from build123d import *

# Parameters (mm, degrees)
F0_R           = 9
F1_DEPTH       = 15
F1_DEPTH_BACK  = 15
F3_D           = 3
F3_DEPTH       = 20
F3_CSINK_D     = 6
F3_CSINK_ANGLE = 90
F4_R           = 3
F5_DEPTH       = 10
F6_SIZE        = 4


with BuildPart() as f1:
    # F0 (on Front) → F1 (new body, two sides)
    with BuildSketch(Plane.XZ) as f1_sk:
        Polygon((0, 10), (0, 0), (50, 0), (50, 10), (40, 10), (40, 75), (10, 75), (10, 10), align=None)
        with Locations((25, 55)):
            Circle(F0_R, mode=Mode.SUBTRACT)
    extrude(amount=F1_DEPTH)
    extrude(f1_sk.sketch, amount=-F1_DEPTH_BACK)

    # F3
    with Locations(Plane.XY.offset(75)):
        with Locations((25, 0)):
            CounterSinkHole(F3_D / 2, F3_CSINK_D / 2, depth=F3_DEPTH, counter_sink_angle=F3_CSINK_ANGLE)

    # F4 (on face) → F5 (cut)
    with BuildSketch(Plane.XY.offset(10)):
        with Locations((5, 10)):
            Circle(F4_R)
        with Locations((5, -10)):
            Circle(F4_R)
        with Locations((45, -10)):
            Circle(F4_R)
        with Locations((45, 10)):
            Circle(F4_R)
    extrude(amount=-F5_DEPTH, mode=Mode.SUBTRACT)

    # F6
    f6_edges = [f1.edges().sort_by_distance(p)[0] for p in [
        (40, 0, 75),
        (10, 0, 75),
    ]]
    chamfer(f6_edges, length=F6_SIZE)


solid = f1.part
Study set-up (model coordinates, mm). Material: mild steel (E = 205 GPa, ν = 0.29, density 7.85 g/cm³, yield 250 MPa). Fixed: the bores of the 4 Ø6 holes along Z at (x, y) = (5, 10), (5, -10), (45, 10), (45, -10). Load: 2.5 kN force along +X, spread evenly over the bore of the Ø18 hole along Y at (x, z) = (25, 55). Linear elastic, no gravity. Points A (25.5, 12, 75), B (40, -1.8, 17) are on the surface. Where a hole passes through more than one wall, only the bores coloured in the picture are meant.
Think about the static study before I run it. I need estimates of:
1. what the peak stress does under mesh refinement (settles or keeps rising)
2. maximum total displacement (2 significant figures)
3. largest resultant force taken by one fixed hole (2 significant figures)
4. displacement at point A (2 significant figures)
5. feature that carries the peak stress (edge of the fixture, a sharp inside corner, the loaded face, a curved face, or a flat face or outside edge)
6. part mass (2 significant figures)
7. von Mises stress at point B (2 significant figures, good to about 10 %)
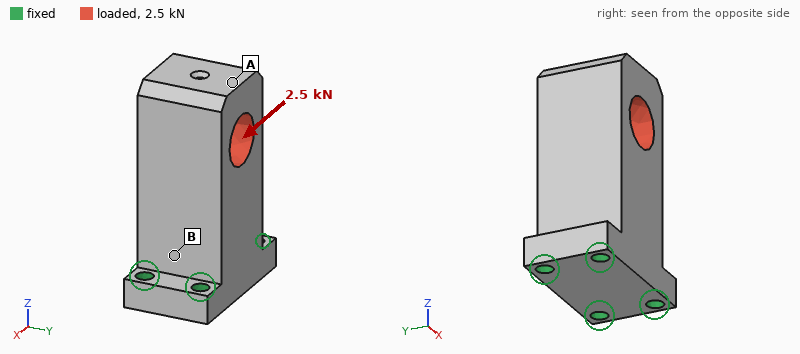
keeps rising
20 µm
2.0 kN
20 µm
edge of the fixture
500 g
22 MPa
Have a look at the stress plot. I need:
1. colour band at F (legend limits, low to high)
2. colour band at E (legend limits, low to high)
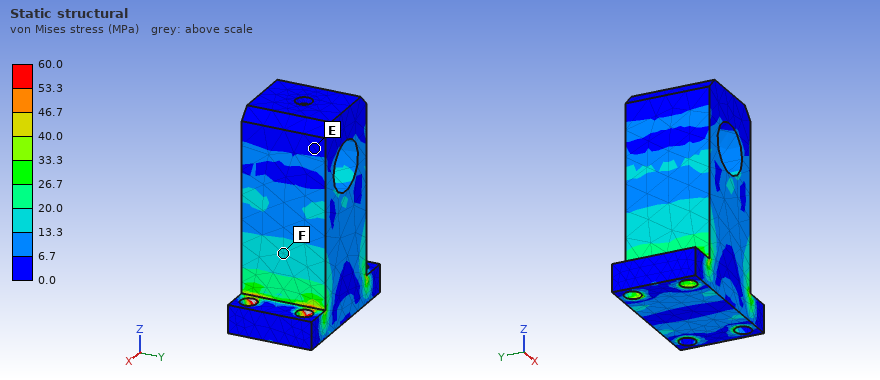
13.3 to 20.0 MPa
0.0 to 6.7 MPa
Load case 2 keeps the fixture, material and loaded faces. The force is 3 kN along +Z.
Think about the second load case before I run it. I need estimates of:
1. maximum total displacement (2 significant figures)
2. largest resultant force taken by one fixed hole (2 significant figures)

2.0 µm
800 N
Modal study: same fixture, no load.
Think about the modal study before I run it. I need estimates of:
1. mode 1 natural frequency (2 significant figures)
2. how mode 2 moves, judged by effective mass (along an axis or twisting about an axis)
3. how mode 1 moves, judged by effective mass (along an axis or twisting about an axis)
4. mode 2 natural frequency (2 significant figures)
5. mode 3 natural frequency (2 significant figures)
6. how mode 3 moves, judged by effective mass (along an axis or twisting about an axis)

3400 Hz
along X
along Y
4300 Hz
10 kHz
twisting about Z
